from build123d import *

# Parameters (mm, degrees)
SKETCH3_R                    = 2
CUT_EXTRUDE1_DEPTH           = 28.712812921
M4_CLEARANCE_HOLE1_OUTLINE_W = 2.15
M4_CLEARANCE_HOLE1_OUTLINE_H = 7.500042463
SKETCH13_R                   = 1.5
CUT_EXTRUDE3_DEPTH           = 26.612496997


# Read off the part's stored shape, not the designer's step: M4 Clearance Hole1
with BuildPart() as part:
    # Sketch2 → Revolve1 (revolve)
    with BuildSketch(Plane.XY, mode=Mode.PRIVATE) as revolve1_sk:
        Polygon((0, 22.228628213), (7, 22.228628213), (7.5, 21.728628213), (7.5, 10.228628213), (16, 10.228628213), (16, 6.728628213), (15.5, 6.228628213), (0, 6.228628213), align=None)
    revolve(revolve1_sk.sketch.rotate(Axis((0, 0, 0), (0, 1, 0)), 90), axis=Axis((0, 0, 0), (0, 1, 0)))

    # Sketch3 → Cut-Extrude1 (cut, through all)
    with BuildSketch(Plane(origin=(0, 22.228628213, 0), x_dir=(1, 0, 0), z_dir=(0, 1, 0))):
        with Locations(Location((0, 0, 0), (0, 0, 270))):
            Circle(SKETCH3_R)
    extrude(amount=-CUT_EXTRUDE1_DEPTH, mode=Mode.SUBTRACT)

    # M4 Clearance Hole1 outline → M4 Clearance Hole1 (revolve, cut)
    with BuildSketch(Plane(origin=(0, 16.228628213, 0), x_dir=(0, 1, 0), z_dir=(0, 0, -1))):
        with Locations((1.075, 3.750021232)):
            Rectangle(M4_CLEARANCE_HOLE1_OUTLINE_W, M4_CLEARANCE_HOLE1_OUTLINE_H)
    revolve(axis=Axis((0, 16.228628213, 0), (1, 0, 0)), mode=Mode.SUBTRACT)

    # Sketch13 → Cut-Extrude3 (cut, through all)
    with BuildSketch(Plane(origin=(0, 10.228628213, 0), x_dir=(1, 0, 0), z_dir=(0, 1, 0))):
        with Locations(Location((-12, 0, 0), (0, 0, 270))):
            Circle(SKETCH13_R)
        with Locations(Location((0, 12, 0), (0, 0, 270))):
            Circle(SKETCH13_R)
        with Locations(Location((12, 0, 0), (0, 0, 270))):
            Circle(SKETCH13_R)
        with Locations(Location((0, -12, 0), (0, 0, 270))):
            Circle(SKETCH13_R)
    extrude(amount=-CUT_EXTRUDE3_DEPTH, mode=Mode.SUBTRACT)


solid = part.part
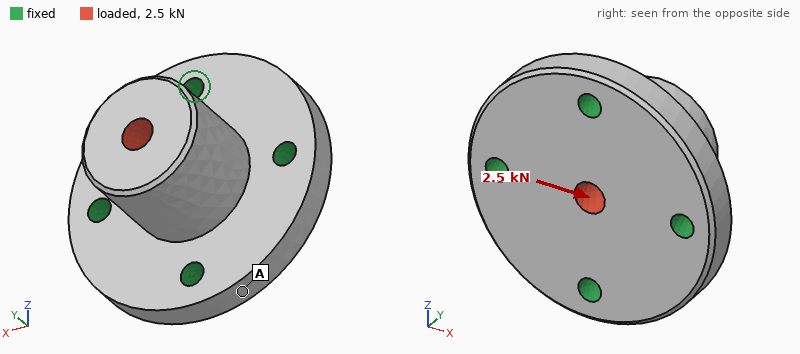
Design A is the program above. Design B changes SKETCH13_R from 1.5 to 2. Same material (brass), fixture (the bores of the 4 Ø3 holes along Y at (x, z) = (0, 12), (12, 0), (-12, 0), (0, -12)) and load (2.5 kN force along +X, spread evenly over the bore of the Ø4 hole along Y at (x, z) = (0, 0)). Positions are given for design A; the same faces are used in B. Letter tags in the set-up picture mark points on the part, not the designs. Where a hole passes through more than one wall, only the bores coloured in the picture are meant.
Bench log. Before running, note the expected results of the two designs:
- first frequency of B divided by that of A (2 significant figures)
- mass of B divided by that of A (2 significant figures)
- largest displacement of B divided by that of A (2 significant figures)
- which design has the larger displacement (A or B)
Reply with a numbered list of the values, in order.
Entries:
1. 1.1
2. 0.98
3. 0.91
4. A
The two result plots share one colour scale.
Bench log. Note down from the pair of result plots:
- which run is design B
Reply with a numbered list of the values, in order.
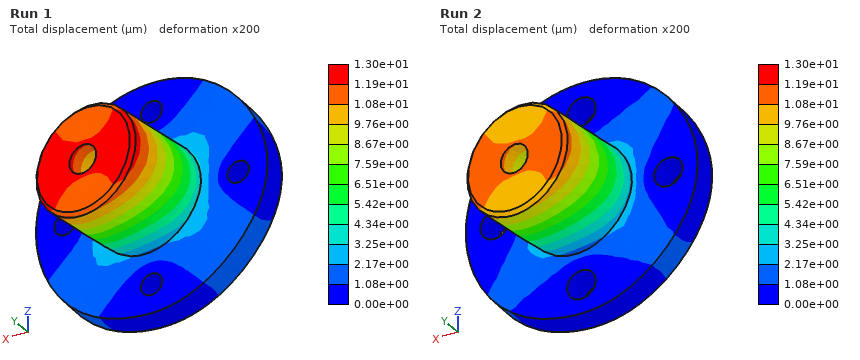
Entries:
1. Run 2
